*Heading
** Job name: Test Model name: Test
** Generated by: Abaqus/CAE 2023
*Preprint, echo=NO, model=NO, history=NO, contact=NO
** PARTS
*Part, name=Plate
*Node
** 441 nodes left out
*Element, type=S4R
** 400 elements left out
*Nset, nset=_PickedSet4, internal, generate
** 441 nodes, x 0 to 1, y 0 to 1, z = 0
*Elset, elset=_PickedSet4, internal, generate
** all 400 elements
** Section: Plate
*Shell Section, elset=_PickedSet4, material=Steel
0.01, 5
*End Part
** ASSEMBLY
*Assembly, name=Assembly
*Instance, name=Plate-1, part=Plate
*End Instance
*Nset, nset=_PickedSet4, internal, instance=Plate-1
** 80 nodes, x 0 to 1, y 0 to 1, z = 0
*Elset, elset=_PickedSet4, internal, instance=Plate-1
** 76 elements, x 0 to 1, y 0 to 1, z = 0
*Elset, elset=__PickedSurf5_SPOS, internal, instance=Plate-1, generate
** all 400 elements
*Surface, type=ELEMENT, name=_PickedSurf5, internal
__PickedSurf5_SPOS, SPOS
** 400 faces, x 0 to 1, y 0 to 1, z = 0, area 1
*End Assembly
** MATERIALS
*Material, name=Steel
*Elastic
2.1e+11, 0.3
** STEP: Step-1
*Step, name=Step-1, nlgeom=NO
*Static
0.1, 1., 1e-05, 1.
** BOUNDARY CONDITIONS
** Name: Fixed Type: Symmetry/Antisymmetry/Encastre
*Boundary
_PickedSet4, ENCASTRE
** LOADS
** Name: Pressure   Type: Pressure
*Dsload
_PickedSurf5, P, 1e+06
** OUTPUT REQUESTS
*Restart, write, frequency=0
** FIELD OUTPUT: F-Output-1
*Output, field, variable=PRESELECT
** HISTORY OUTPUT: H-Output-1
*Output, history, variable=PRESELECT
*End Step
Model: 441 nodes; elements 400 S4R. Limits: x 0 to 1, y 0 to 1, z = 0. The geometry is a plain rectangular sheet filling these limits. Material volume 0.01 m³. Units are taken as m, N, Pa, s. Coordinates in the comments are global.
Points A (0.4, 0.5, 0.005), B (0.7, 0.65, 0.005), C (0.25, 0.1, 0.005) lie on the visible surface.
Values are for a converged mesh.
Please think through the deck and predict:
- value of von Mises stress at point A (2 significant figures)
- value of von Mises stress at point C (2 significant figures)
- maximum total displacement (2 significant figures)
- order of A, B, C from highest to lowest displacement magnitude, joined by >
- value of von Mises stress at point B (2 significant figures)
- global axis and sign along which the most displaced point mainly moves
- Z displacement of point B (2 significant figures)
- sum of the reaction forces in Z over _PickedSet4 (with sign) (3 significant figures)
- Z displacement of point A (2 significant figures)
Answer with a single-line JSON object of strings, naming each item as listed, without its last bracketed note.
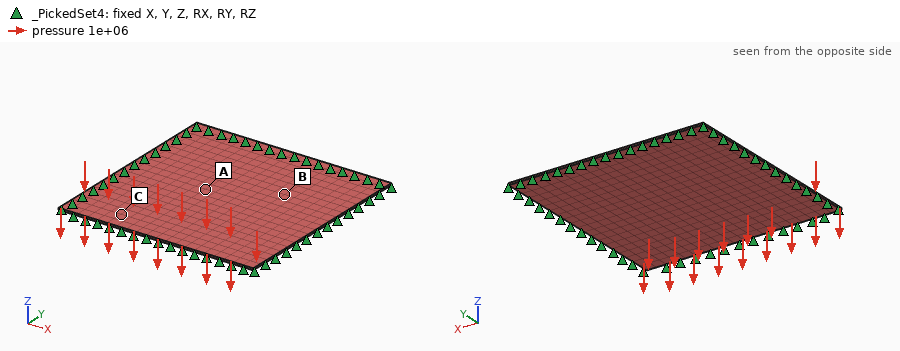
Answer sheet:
{"value of von Mises stress at point A": "1.3e+09 Pa", "value of von Mises stress at point C": "8.6e+08 Pa", "maximum total displacement": "0.065 m", "order of A, B, C from highest to lowest displacement magnitude, joined by >": "A > B > C", "value of von Mises stress at point B": "9.4e+08 Pa", "global axis and sign along which the most displaced point mainly moves": "-Z", "Z displacement of point B": "-0.041 m", "sum of the reaction forces in Z over _PickedSet4 (with sign)": "1.00e+06 N", "Z displacement of point A": "-0.061 m"}
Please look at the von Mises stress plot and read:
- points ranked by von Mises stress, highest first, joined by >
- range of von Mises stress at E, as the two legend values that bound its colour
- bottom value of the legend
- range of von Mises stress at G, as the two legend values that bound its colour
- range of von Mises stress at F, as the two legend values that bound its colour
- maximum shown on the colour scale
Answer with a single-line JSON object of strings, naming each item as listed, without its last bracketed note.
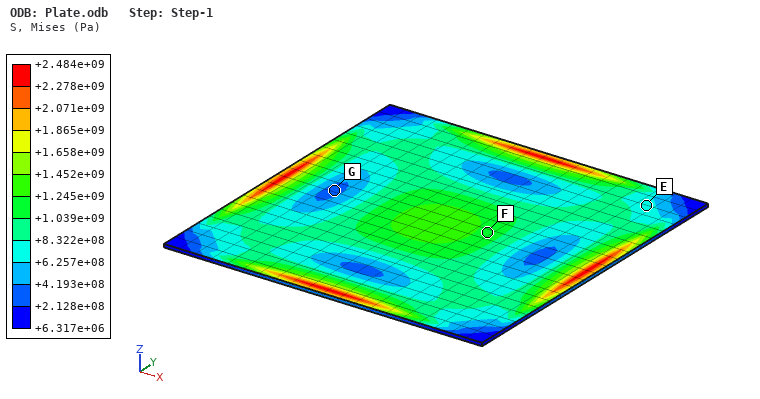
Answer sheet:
{"points ranked by von Mises stress, highest first, joined by >": "F > E > G", "range of von Mises stress at E, as the two legend values that bound its colour": "+6.257e+08 to +8.322e+08 Pa", "bottom value of the legend": "+6.317e+06 Pa", "range of von Mises stress at G, as the two legend values that bound its colour": "+2.128e+08 to +4.193e+08 Pa", "range of von Mises stress at F, as the two legend values that bound its colour": "+1.039e+09 to +1.245e+09 Pa", "maximum shown on the colour scale": "+2.484e+09 Pa"}
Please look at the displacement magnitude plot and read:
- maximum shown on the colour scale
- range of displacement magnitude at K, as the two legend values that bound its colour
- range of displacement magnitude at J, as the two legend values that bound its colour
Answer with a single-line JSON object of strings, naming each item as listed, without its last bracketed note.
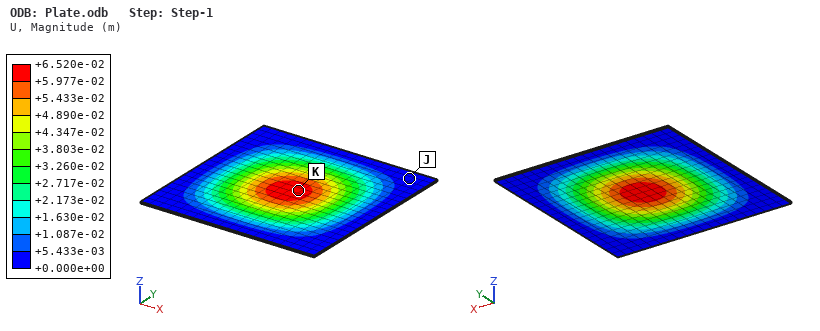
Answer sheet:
{"maximum shown on the colour scale": "+6.520e-02 m", "range of displacement magnitude at K, as the two legend values that bound its colour": "+5.977e-02 to +6.520e-02 m", "range of displacement magnitude at J, as the two legend values that bound its colour": "+0.000e+00 to +5.433e-03 m"}
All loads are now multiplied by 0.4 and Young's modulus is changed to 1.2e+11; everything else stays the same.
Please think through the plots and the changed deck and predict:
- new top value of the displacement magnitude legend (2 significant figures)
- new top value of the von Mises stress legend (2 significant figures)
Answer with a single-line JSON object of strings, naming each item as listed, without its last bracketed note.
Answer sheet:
{"new top value of the displacement magnitude legend": "0.046 m", "new top value of the von Mises stress legend": "9.9e+08 Pa"}
